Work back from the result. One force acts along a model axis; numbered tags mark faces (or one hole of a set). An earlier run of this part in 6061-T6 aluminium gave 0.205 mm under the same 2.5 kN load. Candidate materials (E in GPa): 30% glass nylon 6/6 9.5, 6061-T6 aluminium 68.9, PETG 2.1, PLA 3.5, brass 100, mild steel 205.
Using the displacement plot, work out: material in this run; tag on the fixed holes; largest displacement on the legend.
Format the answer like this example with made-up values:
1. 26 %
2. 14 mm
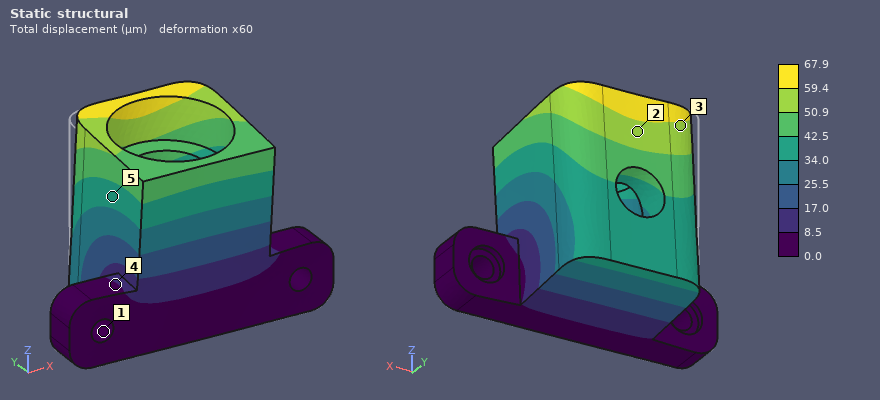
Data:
1. mild steel
2. 1
3. 67.9 µm
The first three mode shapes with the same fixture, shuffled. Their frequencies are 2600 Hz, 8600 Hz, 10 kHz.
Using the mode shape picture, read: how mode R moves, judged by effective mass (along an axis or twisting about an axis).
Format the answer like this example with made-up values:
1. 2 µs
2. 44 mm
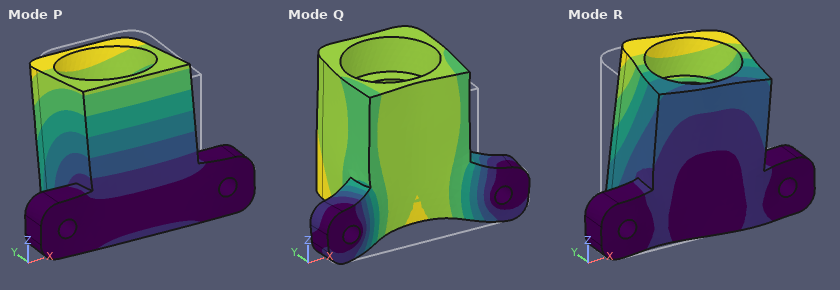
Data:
1. along X
